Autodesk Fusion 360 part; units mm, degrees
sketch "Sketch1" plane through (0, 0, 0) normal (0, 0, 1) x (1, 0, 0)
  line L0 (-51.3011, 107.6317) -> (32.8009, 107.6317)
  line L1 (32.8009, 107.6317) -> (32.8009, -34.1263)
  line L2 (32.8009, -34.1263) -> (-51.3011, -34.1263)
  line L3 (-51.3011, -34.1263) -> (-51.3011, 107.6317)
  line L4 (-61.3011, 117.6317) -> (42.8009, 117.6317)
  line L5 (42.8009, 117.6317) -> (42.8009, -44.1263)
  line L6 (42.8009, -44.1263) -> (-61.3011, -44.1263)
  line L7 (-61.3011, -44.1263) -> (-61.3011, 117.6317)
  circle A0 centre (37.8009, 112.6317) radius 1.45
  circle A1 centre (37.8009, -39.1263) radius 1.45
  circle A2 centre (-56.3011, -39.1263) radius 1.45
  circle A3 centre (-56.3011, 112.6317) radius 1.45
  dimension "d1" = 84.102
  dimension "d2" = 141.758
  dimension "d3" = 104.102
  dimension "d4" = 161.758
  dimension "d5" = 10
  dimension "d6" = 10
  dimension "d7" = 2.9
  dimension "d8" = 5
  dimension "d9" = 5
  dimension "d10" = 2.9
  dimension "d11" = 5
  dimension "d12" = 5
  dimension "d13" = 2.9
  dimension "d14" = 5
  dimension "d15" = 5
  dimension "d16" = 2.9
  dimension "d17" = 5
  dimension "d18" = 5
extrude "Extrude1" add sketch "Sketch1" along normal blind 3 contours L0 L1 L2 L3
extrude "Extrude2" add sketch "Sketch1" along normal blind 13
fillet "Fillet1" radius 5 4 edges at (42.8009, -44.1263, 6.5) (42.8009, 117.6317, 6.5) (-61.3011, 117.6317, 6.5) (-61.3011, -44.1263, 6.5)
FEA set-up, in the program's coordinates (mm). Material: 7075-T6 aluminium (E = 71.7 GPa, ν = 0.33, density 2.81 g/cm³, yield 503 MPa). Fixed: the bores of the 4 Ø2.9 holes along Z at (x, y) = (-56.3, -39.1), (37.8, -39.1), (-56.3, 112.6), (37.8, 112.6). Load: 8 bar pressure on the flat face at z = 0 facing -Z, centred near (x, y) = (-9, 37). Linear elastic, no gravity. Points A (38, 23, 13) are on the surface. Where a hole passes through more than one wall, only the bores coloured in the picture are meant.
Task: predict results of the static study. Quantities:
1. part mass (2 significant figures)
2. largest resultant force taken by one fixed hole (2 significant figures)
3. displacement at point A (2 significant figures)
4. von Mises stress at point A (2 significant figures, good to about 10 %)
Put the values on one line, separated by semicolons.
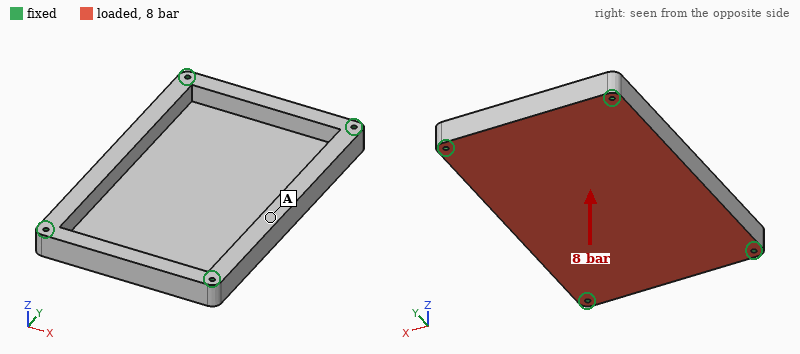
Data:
280 g; 4.4 kN; 0.36 mm; 100 MPa
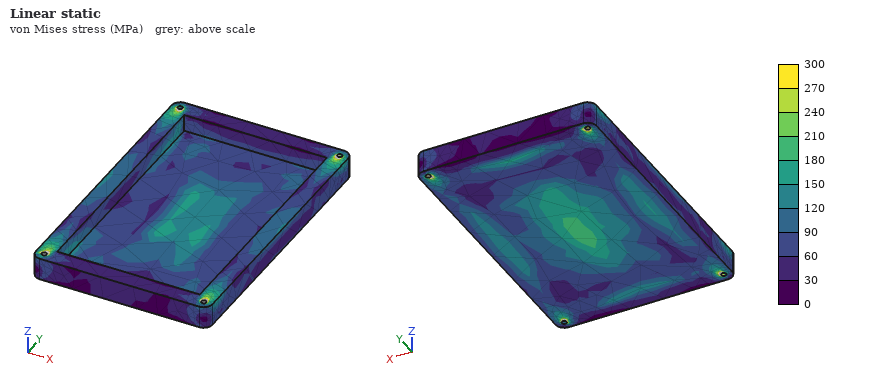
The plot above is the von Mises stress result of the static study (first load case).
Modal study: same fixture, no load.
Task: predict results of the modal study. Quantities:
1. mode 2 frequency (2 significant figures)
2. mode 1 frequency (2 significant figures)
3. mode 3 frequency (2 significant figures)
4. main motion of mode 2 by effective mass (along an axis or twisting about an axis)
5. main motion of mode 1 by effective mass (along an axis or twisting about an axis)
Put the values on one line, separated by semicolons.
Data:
2600 Hz; 1800 Hz; 3300 Hz; twisting about Y; along Z
